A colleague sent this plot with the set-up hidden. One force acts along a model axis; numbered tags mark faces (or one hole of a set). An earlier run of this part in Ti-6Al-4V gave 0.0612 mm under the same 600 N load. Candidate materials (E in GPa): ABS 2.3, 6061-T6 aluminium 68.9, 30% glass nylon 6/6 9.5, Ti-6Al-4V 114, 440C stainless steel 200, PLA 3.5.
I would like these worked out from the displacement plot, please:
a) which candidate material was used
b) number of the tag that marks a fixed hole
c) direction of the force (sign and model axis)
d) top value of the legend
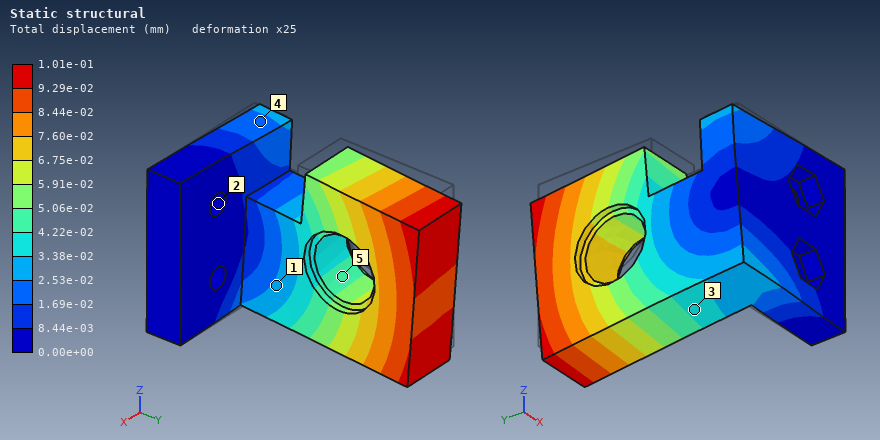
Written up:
6061-T6 aluminium
2
-Z
1.01e-01 mm
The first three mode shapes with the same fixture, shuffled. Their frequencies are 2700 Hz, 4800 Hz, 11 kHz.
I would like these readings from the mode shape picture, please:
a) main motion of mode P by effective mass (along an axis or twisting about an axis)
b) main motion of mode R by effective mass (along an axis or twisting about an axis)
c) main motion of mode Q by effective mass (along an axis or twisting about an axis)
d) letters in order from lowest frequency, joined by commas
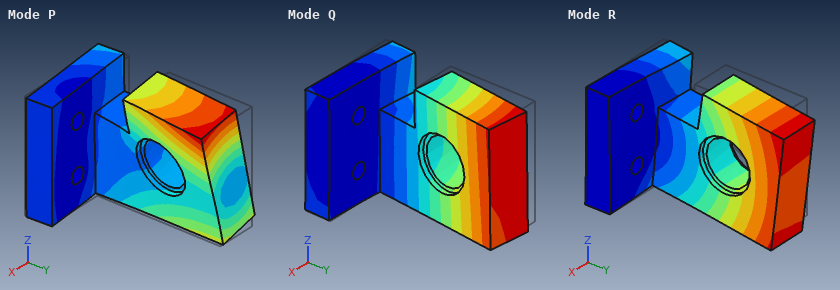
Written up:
along Y
along Z
along X
Q, R, P
